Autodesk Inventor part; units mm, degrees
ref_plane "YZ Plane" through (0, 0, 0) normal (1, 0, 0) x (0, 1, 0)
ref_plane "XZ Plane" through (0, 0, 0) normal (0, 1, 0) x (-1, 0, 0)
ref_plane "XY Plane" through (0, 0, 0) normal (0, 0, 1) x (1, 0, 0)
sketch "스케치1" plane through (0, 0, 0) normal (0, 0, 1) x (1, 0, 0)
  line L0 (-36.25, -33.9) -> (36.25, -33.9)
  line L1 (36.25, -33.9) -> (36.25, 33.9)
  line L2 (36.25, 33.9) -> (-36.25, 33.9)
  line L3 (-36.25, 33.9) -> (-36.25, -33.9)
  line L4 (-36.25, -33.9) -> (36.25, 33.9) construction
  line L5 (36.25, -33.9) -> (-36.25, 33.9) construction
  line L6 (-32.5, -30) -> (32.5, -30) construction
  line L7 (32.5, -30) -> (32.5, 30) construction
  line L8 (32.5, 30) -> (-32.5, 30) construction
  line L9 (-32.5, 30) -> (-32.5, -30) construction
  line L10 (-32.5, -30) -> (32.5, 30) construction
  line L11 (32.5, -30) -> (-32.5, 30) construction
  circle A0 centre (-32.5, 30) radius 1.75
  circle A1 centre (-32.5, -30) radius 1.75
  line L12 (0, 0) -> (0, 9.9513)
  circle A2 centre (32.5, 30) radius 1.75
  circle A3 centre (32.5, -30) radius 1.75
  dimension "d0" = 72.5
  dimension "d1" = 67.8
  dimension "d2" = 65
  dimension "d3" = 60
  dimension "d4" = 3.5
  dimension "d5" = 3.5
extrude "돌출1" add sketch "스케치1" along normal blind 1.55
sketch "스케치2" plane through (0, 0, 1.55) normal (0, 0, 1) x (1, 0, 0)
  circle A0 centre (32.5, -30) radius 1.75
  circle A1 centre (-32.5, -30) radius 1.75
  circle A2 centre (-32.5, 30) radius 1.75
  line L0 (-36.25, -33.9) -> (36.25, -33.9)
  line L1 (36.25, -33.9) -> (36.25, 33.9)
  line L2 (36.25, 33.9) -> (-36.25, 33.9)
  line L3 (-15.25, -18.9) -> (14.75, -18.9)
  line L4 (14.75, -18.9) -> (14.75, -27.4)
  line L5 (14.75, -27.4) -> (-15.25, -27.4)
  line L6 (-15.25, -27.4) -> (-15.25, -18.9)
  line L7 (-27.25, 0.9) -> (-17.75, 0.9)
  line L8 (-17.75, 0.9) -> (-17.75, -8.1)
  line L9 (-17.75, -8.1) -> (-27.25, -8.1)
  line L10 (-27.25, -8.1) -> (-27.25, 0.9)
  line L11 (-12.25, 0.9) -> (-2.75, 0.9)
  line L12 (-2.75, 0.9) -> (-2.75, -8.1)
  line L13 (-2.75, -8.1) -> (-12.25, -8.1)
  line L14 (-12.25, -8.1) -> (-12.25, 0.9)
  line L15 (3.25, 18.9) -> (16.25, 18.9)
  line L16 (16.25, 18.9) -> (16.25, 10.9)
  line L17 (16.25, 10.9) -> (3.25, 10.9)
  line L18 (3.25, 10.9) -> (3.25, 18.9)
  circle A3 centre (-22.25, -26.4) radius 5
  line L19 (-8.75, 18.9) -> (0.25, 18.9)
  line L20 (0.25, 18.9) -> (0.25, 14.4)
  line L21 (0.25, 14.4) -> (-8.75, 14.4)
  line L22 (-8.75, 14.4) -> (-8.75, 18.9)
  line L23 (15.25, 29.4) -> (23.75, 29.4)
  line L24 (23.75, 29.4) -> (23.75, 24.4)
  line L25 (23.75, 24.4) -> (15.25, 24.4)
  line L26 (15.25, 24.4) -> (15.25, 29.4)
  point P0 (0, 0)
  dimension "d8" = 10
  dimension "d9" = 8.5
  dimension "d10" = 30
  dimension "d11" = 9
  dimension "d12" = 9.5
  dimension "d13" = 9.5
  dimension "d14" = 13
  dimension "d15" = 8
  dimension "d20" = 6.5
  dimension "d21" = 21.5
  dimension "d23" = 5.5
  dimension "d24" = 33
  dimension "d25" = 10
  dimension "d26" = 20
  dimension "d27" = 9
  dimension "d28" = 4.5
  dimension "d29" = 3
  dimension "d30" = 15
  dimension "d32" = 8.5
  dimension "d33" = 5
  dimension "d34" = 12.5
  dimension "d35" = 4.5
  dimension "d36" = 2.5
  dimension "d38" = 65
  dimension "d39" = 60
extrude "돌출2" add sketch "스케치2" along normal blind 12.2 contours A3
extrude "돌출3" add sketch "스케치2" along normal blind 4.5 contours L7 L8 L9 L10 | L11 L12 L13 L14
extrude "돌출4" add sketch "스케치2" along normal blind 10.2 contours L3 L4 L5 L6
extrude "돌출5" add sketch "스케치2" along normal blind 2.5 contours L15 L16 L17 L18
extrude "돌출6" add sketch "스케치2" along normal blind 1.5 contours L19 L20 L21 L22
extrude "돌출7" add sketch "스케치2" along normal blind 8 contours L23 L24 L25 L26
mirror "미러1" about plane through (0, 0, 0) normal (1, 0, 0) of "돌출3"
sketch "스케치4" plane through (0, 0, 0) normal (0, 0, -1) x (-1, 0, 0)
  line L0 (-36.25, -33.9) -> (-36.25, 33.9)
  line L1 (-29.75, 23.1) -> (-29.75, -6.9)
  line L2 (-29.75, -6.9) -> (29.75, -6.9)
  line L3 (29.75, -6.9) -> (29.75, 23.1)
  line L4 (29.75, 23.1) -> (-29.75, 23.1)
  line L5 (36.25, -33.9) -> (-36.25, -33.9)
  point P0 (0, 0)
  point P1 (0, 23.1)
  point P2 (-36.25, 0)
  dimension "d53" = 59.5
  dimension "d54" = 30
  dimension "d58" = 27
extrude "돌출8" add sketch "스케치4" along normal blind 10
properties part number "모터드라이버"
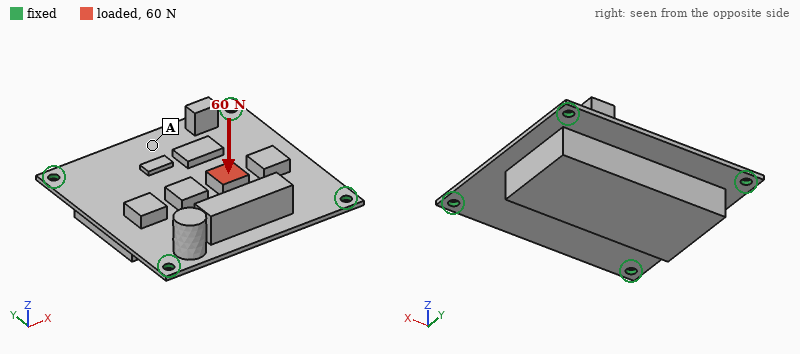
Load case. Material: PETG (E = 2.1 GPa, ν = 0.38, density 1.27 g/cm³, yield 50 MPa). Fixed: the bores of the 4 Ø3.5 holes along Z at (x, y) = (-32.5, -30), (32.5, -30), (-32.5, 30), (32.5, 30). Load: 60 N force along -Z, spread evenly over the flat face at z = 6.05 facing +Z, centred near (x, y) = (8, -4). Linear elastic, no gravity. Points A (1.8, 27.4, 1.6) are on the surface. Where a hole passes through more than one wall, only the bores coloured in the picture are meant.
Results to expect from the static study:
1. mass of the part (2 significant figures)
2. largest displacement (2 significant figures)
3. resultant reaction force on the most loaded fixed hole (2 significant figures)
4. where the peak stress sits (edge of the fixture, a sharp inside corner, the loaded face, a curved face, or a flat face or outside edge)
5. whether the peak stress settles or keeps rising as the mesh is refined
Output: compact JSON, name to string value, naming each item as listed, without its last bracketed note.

{"mass of the part": "40 g", "largest displacement": "0.92 mm", "resultant reaction force on the most loaded fixed hole": "22 N", "where the peak stress sits": "edge of the fixture", "whether the peak stress settles or keeps rising as the mesh is refined": "keeps rising"}
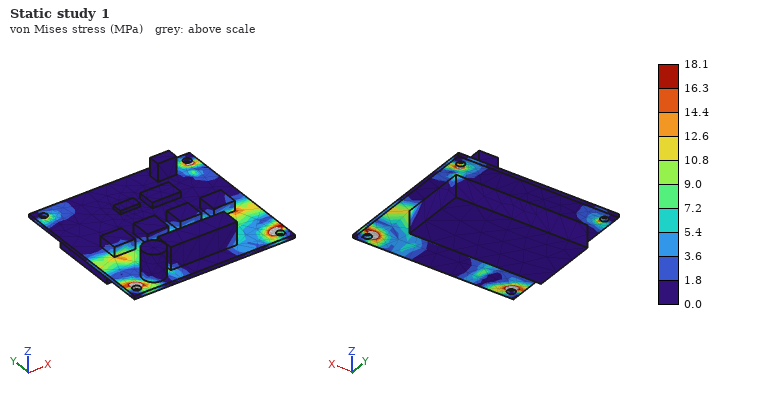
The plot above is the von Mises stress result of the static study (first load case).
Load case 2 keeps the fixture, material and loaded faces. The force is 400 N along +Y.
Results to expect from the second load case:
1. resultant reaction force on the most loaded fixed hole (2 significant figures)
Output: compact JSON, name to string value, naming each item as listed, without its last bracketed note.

{"resultant reaction force on the most loaded fixed hole": "130 N"}
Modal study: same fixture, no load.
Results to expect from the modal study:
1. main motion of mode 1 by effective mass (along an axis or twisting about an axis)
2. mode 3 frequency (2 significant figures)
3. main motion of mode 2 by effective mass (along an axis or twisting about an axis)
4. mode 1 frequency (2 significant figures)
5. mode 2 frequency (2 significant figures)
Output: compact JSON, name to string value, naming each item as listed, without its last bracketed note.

{"main motion of mode 1 by effective mass": "along Z", "mode 3 frequency": "810 Hz", "main motion of mode 2 by effective mass": "twisting about X", "mode 1 frequency": "300 Hz", "mode 2 frequency": "660 Hz"}
